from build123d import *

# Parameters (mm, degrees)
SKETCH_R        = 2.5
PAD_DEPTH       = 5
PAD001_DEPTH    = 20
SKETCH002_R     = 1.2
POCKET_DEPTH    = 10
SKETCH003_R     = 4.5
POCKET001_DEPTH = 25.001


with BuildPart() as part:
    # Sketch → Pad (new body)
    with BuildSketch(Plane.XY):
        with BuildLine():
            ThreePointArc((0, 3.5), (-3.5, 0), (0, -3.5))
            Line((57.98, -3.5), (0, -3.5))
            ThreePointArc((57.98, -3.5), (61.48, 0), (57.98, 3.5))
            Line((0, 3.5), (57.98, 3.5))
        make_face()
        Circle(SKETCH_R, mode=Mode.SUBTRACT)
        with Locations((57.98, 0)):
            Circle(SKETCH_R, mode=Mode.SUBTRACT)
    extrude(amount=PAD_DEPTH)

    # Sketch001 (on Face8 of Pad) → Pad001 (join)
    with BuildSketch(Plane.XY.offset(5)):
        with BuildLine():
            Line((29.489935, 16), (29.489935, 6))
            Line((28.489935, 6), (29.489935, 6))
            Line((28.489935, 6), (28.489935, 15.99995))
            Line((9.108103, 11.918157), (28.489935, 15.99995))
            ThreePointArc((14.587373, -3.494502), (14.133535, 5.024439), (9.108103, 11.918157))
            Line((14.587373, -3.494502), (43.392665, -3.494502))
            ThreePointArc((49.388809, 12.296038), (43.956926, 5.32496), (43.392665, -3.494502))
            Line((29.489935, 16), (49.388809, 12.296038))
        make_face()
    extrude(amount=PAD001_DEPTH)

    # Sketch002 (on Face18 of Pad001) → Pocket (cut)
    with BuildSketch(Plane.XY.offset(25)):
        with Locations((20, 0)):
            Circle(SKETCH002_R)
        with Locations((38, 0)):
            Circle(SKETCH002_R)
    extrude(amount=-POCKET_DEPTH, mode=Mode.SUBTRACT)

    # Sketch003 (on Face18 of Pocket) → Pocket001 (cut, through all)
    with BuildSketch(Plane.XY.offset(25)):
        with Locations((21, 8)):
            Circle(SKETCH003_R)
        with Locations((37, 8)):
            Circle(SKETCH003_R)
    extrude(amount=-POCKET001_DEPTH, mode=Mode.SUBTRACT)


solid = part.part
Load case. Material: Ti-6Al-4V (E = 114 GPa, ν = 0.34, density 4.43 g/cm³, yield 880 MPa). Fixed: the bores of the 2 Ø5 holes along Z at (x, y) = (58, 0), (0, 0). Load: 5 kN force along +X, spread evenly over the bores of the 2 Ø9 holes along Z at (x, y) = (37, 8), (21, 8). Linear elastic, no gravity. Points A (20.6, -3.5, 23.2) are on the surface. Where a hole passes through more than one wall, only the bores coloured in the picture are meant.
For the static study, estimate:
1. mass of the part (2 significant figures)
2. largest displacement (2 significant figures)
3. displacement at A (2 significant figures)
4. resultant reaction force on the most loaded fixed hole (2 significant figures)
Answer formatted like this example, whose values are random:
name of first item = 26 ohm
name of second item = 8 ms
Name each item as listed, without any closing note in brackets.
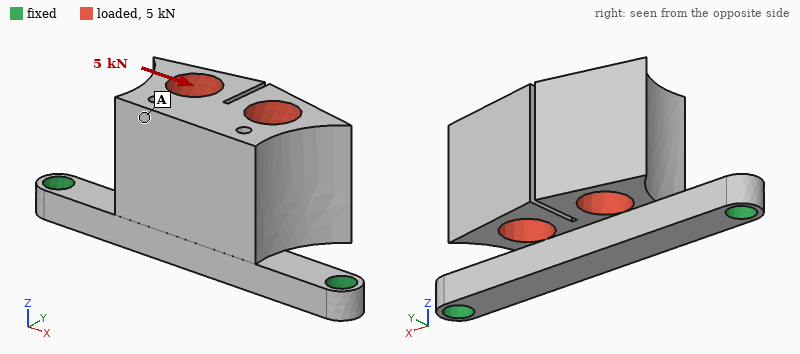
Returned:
mass of the part = 46 g
largest displacement = 0.15 mm
displacement at A = 0.078 mm
resultant reaction force on the most loaded fixed hole = 3.1 kN
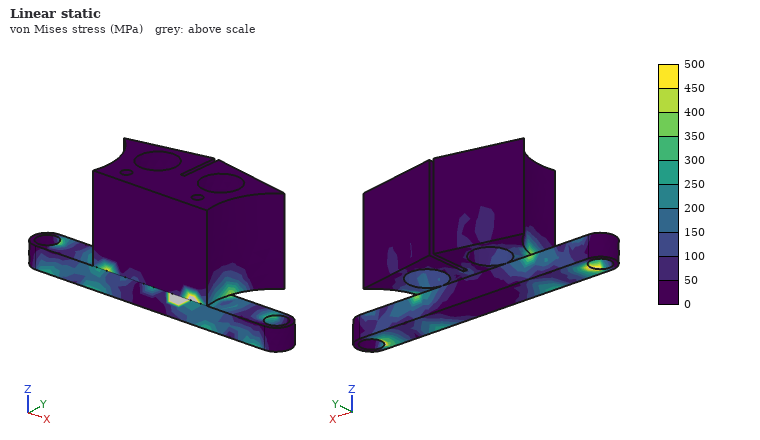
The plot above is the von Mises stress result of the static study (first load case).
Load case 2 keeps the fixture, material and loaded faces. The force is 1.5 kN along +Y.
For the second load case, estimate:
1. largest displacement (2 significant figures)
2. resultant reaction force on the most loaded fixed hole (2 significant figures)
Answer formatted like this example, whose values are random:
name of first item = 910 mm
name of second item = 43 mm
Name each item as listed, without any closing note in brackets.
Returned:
largest displacement = 0.57 mm
resultant reaction force on the most loaded fixed hole = 750 N
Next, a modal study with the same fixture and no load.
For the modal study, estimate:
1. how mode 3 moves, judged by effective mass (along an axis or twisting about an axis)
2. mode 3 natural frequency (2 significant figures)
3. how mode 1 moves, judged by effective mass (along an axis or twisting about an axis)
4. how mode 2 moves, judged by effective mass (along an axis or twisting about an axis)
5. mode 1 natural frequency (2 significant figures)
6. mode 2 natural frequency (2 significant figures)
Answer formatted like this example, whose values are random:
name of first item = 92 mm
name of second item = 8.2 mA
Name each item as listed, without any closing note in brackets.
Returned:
how mode 3 moves, judged by effective mass = along X
mode 3 natural frequency = 6000 Hz
how mode 1 moves, judged by effective mass = along Y
how mode 2 moves, judged by effective mass = along Z
mode 1 natural frequency = 1600 Hz
mode 2 natural frequency = 5000 Hz
